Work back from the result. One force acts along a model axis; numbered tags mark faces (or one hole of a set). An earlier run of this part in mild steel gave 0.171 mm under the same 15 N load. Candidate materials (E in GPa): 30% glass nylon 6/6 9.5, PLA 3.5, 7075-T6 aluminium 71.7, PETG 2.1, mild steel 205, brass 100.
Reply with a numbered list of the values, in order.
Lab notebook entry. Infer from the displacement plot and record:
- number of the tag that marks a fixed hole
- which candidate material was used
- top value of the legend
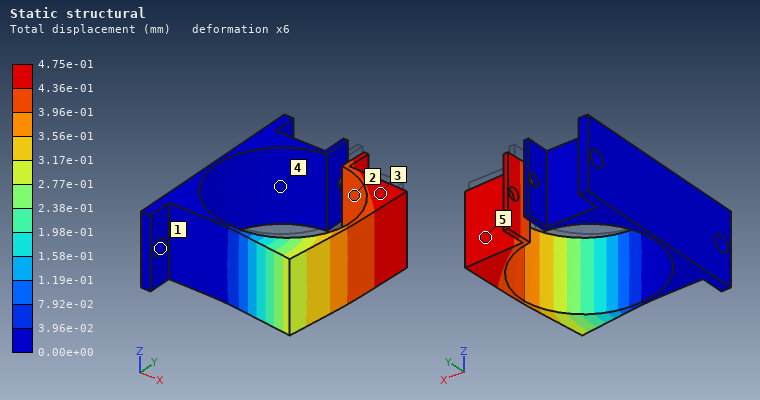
1. 1
2. 7075-T6 aluminium
3. 4.75e-01 mm
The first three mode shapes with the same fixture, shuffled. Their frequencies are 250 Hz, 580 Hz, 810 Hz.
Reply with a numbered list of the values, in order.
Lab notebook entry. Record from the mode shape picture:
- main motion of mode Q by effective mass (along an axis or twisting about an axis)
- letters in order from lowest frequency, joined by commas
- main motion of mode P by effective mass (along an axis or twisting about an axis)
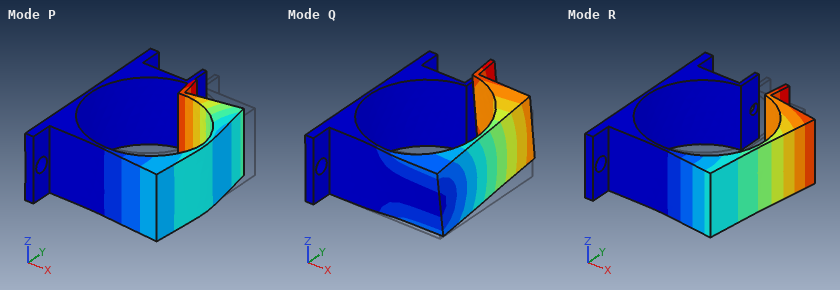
1. along Z
2. R, Q, P
3. along Y
